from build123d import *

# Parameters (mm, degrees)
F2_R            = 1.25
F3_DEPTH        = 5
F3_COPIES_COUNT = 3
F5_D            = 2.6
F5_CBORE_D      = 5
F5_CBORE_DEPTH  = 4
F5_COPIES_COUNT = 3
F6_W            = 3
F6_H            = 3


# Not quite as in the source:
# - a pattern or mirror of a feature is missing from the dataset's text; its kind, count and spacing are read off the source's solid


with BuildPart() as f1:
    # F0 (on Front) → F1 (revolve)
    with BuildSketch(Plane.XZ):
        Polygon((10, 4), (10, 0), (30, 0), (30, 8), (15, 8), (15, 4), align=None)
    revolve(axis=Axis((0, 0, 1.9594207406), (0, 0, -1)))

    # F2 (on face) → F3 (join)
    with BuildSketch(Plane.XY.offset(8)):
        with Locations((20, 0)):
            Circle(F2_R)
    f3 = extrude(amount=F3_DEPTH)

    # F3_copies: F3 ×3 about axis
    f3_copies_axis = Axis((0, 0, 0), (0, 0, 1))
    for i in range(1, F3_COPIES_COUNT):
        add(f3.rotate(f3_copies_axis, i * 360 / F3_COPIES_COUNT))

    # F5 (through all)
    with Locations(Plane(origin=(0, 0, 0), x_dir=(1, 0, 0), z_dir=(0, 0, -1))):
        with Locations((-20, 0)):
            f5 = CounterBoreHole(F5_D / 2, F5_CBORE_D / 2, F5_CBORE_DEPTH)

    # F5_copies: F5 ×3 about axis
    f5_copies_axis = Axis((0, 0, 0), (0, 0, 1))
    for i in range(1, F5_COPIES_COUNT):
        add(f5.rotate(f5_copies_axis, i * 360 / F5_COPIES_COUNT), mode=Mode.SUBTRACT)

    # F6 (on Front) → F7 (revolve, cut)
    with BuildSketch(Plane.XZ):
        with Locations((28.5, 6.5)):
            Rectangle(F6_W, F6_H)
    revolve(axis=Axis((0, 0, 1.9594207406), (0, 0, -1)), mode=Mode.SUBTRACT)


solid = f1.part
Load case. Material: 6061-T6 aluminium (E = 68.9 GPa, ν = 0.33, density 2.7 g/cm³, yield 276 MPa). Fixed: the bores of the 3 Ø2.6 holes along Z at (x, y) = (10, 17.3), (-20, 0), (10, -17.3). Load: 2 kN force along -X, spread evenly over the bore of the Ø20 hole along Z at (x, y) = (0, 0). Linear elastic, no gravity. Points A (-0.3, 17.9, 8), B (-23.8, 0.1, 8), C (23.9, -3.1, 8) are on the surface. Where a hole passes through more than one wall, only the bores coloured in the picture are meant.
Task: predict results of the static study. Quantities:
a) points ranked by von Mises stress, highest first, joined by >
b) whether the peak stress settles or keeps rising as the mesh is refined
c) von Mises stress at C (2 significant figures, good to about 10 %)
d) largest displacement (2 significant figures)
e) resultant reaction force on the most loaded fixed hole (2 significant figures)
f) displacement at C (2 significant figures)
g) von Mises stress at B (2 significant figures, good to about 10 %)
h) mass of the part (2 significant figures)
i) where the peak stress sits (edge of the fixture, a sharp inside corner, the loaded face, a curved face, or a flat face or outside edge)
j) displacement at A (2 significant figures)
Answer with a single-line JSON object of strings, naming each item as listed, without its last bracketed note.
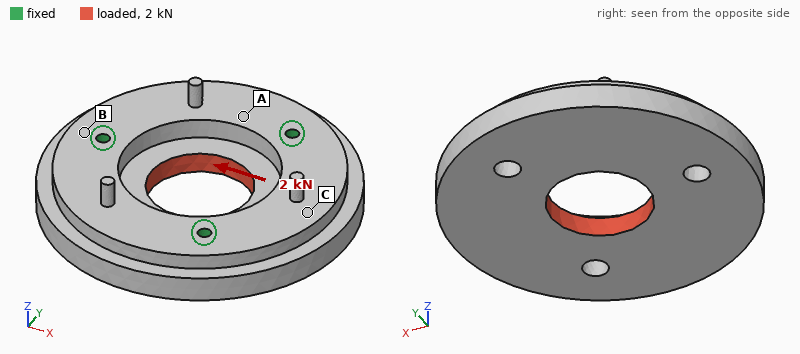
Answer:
{"points ranked by von Mises stress, highest first, joined by >": "B > A > C", "whether the peak stress settles or keeps rising as the mesh is refined": "keeps rising", "von Mises stress at C": "3.8 MPa", "largest displacement": "12 µm", "resultant reaction force on the most loaded fixed hole": "700 N", "displacement at C": "7.3 µm", "von Mises stress at B": "13 MPa", "mass of the part": "45 g", "where the peak stress sits": "edge of the fixture", "displacement at A": "2.2 µm"}
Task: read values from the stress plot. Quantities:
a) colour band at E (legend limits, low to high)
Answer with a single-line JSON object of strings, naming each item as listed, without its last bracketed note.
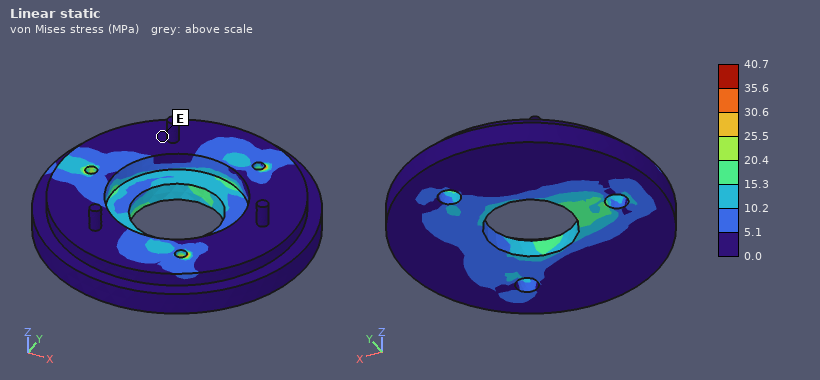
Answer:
{"colour band at E": "0.0 to 5.1 MPa"}
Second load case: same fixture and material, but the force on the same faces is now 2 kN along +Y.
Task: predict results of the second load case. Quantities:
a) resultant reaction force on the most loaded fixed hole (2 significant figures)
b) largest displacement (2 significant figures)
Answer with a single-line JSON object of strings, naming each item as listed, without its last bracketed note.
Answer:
{"resultant reaction force on the most loaded fixed hole": "710 N", "largest displacement": "10 µm"}
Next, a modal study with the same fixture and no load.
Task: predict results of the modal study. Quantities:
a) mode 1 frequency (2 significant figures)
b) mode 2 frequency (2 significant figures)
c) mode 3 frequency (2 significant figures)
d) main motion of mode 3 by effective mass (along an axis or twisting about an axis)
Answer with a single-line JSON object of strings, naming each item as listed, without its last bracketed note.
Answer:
{"mode 1 frequency": "8500 Hz", "mode 2 frequency": "8500 Hz", "mode 3 frequency": "13 kHz", "main motion of mode 3 by effective mass": "along Z"}
